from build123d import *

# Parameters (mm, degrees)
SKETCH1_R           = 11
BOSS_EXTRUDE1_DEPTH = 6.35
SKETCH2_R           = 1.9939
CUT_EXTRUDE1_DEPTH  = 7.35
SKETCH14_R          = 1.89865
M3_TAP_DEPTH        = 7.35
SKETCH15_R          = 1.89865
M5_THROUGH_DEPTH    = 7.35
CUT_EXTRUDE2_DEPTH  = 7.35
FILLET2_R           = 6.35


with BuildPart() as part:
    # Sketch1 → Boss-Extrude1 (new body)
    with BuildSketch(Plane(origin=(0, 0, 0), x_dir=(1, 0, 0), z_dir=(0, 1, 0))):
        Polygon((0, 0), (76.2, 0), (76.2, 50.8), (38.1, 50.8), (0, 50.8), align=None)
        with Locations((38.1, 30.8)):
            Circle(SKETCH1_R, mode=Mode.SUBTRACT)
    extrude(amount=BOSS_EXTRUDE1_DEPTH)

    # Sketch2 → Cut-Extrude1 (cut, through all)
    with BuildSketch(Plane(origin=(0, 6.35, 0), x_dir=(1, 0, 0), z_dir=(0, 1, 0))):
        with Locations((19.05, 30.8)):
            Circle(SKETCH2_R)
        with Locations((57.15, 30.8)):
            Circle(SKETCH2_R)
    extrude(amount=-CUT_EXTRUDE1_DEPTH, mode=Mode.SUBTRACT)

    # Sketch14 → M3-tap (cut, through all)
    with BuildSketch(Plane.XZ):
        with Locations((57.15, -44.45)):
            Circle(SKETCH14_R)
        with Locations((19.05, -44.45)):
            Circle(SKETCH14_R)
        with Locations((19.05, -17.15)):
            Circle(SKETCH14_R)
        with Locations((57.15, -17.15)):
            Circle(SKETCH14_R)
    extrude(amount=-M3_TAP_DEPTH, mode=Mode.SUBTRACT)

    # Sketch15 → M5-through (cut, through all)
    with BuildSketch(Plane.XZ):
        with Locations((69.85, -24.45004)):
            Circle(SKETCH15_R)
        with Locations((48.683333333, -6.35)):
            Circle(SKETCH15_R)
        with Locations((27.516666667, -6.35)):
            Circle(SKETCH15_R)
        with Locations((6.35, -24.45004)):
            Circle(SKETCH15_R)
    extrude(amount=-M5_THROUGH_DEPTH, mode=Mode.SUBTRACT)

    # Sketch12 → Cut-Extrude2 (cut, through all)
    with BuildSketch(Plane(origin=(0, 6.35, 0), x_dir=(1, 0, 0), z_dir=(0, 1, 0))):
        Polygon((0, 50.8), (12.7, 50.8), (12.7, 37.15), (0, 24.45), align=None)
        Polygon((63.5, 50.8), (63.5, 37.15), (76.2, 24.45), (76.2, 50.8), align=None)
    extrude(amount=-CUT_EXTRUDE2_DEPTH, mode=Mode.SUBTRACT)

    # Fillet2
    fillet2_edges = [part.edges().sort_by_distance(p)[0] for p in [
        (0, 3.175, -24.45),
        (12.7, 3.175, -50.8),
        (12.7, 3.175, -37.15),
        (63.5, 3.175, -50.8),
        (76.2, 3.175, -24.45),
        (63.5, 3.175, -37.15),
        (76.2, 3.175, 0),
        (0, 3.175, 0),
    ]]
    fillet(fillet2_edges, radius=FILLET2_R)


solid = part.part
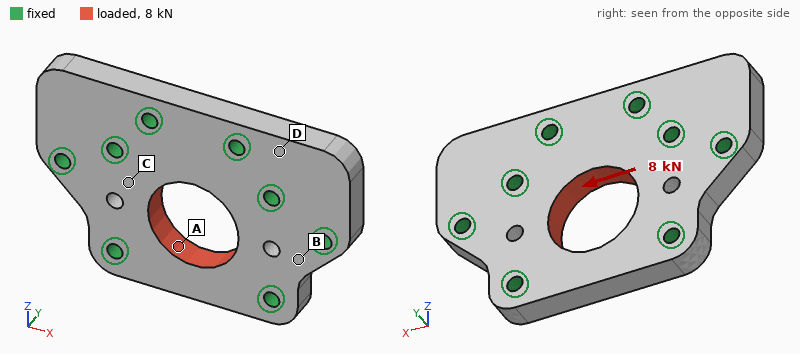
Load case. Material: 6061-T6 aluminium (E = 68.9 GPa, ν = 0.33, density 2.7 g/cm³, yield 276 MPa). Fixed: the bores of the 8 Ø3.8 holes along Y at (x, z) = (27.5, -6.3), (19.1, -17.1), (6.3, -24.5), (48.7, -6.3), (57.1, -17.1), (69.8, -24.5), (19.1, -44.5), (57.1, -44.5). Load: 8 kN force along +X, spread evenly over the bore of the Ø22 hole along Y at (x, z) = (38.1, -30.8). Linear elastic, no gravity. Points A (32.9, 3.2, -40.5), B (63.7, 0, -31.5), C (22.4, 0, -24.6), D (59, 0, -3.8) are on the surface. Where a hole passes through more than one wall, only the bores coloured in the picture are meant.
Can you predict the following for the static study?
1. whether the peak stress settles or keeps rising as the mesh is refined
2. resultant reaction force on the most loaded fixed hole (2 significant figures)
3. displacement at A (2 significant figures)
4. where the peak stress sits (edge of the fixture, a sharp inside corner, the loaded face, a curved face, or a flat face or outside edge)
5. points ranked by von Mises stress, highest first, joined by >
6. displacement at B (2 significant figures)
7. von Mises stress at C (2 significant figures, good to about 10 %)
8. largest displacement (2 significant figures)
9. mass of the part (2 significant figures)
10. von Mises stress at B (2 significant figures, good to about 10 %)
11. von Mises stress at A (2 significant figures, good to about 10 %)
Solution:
keeps rising
1.8 kN
4.8 µm
edge of the fixture
A > C > B > D
2.1 µm
16 MPa
5.4 µm
49 g
10 MPa
30 MPa
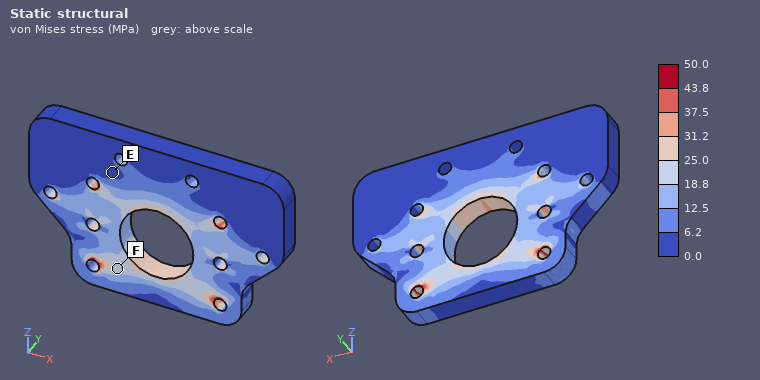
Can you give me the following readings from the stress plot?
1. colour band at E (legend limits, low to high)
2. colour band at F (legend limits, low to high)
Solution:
0.0 to 6.2 MPa
18.8 to 25.0 MPa
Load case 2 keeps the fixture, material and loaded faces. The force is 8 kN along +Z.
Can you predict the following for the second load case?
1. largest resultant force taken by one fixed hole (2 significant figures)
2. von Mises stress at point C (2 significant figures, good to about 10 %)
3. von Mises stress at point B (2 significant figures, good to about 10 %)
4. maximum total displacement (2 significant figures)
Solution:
1.5 kN
24 MPa
9.9 MPa
16 µm
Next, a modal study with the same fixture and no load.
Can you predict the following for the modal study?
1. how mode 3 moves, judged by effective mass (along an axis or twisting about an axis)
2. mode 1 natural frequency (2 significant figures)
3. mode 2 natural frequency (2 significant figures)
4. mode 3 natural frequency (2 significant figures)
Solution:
along Y
16 kHz
16 kHz
22 kHz
